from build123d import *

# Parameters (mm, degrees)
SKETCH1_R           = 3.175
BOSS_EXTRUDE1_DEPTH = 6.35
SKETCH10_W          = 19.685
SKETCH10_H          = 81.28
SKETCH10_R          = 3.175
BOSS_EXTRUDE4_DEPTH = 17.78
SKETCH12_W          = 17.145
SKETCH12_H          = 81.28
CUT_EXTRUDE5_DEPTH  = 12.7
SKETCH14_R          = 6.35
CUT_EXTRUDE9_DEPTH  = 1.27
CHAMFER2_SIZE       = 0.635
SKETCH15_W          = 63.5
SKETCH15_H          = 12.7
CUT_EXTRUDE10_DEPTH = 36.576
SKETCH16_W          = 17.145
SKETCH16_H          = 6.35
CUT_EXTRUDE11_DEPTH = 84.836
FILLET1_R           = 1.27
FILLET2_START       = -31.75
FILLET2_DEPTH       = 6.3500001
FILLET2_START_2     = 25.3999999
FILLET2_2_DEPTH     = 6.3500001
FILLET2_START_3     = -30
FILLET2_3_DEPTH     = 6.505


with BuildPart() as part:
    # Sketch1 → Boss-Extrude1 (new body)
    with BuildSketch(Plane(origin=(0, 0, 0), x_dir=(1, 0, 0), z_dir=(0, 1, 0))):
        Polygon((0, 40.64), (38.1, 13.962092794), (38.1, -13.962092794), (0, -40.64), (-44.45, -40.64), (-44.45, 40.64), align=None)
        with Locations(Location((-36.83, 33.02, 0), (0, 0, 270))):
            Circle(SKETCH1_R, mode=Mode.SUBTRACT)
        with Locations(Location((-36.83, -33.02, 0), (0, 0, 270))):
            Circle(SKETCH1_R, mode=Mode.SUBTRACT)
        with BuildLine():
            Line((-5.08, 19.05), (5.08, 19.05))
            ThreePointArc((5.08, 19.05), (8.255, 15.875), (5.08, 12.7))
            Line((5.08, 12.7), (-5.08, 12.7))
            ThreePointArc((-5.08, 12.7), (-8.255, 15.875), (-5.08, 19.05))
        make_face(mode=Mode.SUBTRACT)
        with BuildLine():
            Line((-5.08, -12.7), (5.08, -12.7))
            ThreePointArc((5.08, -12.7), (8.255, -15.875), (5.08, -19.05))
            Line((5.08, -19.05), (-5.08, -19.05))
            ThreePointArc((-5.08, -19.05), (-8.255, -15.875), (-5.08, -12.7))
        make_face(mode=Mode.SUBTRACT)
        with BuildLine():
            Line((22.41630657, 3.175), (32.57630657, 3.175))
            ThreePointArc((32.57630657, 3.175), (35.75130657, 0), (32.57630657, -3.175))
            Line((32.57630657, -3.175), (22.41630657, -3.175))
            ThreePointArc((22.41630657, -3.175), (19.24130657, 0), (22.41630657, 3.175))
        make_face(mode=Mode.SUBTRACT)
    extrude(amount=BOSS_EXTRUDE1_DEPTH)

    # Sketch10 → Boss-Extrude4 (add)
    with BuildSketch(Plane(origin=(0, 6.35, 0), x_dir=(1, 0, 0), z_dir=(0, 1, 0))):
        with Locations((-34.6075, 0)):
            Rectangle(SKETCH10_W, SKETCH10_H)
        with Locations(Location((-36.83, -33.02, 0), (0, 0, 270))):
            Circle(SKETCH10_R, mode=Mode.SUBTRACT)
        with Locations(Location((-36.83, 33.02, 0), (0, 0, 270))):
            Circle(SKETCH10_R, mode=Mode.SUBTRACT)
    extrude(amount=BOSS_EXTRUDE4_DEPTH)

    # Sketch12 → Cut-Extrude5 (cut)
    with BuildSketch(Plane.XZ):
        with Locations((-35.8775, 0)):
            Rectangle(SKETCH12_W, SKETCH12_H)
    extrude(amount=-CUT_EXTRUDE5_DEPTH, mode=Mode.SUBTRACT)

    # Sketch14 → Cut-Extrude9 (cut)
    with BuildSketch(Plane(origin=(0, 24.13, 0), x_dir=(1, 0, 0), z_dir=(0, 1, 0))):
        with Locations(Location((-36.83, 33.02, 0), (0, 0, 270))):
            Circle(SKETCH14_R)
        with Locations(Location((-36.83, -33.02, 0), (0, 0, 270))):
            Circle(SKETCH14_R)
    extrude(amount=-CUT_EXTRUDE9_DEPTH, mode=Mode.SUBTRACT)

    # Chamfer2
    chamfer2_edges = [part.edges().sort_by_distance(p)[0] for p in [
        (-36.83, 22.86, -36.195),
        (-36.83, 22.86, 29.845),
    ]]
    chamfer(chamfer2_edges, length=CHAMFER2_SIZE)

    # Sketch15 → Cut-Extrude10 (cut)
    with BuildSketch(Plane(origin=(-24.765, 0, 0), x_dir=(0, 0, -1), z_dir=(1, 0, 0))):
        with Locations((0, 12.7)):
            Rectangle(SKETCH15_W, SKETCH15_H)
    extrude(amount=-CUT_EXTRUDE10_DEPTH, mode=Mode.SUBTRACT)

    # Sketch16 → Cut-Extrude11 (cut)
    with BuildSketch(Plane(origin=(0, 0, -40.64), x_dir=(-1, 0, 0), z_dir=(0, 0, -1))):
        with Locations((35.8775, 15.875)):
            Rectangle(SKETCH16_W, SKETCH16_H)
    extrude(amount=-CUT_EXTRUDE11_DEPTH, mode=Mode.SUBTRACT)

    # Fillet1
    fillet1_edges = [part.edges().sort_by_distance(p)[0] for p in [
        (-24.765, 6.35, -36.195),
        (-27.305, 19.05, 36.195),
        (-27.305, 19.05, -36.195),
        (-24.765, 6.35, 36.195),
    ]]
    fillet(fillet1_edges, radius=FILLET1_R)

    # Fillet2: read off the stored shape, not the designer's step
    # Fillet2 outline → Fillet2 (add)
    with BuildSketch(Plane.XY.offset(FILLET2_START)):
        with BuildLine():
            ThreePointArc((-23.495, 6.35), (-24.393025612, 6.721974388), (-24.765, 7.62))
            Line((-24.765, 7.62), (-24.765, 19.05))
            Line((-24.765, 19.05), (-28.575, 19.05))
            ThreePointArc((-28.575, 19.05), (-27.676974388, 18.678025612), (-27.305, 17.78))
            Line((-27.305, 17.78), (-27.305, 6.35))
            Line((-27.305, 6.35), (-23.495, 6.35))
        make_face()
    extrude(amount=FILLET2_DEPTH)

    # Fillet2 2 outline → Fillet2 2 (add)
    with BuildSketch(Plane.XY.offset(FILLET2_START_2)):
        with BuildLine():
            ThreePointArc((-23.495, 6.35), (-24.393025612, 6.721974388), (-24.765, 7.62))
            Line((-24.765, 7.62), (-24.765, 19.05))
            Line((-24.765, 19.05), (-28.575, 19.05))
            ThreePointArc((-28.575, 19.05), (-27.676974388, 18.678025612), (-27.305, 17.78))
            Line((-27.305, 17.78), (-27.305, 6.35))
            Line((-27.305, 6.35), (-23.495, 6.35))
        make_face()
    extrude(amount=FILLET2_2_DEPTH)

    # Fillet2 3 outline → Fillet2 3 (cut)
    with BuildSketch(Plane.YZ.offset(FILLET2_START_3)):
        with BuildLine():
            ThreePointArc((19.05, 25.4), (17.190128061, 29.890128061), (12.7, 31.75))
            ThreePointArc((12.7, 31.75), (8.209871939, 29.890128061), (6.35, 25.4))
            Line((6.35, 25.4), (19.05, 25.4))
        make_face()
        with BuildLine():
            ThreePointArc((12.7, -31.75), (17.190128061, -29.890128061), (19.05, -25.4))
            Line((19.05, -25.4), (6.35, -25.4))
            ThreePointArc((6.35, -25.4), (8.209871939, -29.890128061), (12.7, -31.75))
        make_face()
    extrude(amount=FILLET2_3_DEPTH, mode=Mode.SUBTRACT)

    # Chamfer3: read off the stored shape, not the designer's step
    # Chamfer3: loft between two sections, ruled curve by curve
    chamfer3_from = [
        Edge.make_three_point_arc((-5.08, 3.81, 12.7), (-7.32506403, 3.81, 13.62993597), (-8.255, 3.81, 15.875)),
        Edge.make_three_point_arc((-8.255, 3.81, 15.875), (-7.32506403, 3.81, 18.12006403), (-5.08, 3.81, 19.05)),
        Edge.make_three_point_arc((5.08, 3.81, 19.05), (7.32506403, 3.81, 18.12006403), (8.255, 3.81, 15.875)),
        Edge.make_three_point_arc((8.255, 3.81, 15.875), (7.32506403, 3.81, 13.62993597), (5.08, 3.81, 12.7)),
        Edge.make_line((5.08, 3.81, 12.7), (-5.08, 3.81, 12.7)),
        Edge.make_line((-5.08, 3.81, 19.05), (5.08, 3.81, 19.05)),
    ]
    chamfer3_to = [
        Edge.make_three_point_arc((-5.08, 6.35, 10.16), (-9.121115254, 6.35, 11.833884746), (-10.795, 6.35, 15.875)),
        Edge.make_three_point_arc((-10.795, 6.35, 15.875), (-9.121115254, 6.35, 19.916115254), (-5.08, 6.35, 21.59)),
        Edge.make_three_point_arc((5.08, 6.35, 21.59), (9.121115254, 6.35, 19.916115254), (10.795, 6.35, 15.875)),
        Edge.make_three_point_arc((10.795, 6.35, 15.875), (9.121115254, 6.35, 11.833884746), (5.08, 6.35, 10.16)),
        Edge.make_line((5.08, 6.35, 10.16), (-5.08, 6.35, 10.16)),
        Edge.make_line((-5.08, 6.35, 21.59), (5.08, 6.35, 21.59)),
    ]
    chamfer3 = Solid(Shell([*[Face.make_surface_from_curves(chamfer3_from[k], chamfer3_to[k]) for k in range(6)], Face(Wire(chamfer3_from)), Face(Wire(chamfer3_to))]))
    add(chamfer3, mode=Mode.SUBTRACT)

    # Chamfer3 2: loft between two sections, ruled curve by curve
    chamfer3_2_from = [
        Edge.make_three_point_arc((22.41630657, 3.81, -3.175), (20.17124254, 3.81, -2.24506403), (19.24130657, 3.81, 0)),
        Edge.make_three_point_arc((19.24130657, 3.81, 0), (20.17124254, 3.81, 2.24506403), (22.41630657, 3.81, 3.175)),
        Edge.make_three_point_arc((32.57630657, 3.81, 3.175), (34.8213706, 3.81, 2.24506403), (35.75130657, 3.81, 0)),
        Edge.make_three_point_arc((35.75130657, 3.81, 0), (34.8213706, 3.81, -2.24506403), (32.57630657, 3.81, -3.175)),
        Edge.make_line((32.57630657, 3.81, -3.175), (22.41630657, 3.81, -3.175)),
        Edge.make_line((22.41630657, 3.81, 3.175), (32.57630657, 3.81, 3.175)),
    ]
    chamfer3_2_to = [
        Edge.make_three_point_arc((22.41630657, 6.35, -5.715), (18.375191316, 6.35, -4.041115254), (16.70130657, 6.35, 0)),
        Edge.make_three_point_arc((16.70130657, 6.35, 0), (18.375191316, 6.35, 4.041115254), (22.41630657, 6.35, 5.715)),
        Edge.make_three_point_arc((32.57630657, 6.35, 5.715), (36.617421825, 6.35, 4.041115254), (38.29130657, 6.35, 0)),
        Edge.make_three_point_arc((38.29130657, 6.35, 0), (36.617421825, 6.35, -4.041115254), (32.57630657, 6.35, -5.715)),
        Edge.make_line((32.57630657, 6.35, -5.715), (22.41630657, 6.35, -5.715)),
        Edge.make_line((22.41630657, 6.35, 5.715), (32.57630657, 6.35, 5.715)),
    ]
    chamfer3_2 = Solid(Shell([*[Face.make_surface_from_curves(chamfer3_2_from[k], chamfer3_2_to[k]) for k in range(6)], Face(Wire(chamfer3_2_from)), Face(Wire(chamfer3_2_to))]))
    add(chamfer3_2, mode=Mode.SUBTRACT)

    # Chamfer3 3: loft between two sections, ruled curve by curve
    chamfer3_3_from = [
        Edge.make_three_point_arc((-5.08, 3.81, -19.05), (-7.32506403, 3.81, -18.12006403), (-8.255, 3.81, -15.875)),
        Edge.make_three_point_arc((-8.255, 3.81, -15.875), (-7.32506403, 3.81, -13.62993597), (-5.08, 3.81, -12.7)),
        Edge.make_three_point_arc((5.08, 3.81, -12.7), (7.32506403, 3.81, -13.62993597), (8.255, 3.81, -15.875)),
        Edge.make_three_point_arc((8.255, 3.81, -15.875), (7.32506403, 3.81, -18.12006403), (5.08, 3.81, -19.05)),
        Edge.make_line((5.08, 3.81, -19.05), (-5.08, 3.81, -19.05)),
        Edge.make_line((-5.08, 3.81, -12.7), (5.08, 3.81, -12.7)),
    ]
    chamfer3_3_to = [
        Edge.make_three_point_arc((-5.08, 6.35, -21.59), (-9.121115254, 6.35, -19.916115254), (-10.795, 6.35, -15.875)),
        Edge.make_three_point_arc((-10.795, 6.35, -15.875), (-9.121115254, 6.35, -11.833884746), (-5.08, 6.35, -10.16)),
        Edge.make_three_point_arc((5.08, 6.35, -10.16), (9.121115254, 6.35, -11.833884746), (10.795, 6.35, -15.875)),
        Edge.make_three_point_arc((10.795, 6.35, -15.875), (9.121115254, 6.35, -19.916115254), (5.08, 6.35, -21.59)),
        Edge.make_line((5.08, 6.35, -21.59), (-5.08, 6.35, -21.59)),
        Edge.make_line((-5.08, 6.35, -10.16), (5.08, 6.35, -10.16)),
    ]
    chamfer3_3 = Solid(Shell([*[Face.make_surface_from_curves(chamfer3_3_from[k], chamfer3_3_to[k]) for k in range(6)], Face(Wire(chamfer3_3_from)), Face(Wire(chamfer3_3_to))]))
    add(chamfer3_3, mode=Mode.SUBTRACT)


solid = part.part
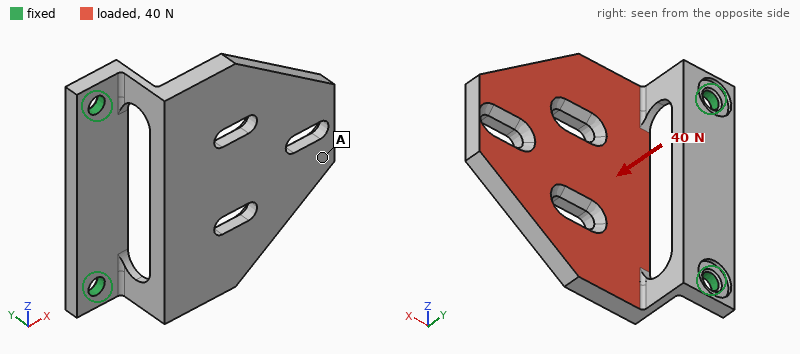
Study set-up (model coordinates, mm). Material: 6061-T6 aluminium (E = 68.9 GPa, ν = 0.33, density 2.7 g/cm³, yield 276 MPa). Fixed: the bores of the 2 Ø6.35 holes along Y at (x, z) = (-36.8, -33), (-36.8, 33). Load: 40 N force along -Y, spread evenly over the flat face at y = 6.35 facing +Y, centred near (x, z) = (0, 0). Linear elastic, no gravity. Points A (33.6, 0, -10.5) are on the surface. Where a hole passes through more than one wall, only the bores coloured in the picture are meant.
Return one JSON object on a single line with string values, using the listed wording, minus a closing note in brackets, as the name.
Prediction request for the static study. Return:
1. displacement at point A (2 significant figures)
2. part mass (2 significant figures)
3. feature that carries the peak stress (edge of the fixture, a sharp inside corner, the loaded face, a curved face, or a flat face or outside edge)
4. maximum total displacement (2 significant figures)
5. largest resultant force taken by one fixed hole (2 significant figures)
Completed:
{"displacement at point A": "0.53 mm", "part mass": "90 g", "feature that carries the peak stress": "a curved face", "maximum total displacement": "0.57 mm", "largest resultant force taken by one fixed hole": "20 N"}
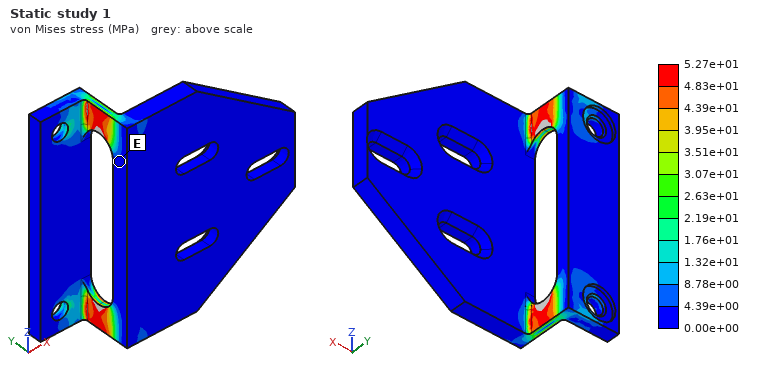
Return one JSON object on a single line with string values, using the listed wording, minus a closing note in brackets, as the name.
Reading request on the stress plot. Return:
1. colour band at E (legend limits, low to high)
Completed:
{"colour band at E": "0.00e+00 to 4.39e+00 MPa"}
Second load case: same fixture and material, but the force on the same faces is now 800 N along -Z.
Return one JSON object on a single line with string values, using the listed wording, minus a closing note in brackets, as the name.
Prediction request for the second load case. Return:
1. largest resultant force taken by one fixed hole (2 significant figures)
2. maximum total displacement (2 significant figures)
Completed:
{"largest resultant force taken by one fixed hole": "560 N", "maximum total displacement": "0.24 mm"}
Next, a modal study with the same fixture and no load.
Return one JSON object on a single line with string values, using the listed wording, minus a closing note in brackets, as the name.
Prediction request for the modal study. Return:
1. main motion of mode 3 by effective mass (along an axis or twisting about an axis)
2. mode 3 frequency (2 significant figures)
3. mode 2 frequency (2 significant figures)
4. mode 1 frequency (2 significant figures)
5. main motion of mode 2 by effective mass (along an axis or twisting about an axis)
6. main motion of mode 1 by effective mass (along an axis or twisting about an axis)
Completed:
{"main motion of mode 3 by effective mass": "along X", "mode 3 frequency": "1500 Hz", "mode 2 frequency": "1300 Hz", "mode 1 frequency": "200 Hz", "main motion of mode 2 by effective mass": "along Z", "main motion of mode 1 by effective mass": "along Y"}
